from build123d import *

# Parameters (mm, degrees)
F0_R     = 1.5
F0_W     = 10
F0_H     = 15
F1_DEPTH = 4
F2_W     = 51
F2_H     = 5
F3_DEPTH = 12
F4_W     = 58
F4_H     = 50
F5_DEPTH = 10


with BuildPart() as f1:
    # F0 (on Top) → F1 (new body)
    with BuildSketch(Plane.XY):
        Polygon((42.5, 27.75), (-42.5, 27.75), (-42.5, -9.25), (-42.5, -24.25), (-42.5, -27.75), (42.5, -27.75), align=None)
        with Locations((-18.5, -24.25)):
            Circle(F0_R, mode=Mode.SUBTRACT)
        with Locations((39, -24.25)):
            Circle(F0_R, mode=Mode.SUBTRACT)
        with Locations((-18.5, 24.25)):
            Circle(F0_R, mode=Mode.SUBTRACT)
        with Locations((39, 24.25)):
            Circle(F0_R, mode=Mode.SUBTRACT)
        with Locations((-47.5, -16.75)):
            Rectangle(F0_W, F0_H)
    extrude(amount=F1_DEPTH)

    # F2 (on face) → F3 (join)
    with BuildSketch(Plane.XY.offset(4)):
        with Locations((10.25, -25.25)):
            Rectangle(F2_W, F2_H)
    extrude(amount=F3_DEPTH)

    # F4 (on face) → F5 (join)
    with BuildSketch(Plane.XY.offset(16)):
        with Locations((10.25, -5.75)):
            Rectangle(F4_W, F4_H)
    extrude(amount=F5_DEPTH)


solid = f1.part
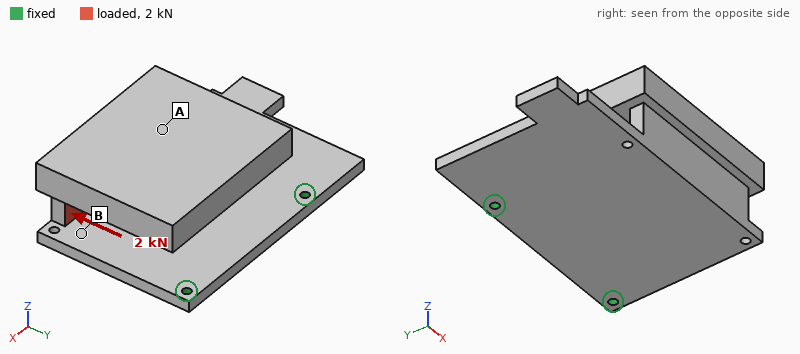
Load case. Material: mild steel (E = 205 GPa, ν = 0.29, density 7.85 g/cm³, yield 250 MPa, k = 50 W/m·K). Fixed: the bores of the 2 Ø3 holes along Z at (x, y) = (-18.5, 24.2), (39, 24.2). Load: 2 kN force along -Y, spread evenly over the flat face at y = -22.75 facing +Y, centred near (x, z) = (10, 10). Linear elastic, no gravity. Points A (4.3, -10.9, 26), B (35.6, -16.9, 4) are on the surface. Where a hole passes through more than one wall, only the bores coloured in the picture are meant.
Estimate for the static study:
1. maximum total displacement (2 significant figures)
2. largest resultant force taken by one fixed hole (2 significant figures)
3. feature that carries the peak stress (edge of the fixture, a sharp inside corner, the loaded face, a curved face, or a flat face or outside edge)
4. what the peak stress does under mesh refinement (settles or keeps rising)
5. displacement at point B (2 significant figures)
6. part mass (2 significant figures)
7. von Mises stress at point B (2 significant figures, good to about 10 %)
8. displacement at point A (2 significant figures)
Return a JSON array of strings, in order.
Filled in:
["0.49 mm", "1.1 kN", "edge of the fixture", "keeps rising", "0.24 mm", "400 g", "77 MPa", "0.32 mm"]
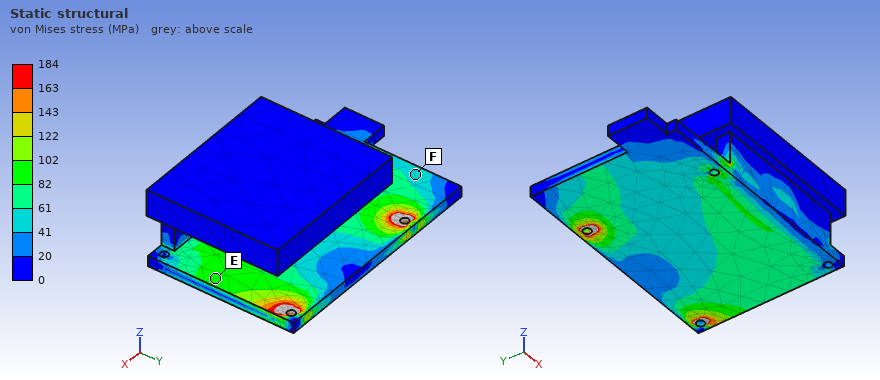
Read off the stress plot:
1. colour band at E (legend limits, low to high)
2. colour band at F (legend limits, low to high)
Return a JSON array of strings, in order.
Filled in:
["82 to 102 MPa", "41 to 61 MPa"]
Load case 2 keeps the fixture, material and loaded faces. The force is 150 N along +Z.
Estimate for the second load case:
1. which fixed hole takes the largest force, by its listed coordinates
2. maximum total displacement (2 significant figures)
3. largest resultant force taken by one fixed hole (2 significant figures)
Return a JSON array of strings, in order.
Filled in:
["(-18.5, 24.2)", "0.14 mm", "80 N"]
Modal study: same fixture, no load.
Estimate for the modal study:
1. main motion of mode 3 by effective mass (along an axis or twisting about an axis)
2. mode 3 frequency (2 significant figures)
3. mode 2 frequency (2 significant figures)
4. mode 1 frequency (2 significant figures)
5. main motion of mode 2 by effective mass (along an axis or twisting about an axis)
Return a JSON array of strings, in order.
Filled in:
["along X", "720 Hz", "660 Hz", "390 Hz", "along Z"]
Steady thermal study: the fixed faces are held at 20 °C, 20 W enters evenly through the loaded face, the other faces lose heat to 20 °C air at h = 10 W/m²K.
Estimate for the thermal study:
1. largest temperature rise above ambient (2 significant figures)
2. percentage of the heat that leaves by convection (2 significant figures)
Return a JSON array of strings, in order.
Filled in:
["64 K", "41 %"]
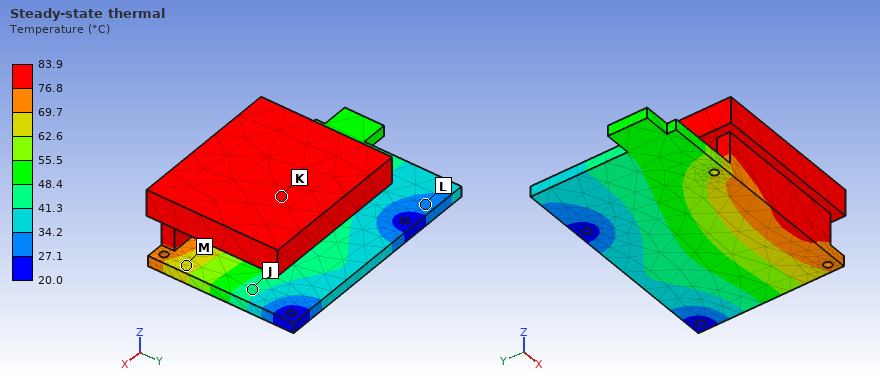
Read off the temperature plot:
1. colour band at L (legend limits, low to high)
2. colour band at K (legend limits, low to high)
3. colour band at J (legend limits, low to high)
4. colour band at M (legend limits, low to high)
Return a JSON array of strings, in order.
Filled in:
["27.1 to 34.2 °C", "76.8 to 83.9 °C", "41.3 to 48.4 °C", "62.6 to 69.7 °C"]
